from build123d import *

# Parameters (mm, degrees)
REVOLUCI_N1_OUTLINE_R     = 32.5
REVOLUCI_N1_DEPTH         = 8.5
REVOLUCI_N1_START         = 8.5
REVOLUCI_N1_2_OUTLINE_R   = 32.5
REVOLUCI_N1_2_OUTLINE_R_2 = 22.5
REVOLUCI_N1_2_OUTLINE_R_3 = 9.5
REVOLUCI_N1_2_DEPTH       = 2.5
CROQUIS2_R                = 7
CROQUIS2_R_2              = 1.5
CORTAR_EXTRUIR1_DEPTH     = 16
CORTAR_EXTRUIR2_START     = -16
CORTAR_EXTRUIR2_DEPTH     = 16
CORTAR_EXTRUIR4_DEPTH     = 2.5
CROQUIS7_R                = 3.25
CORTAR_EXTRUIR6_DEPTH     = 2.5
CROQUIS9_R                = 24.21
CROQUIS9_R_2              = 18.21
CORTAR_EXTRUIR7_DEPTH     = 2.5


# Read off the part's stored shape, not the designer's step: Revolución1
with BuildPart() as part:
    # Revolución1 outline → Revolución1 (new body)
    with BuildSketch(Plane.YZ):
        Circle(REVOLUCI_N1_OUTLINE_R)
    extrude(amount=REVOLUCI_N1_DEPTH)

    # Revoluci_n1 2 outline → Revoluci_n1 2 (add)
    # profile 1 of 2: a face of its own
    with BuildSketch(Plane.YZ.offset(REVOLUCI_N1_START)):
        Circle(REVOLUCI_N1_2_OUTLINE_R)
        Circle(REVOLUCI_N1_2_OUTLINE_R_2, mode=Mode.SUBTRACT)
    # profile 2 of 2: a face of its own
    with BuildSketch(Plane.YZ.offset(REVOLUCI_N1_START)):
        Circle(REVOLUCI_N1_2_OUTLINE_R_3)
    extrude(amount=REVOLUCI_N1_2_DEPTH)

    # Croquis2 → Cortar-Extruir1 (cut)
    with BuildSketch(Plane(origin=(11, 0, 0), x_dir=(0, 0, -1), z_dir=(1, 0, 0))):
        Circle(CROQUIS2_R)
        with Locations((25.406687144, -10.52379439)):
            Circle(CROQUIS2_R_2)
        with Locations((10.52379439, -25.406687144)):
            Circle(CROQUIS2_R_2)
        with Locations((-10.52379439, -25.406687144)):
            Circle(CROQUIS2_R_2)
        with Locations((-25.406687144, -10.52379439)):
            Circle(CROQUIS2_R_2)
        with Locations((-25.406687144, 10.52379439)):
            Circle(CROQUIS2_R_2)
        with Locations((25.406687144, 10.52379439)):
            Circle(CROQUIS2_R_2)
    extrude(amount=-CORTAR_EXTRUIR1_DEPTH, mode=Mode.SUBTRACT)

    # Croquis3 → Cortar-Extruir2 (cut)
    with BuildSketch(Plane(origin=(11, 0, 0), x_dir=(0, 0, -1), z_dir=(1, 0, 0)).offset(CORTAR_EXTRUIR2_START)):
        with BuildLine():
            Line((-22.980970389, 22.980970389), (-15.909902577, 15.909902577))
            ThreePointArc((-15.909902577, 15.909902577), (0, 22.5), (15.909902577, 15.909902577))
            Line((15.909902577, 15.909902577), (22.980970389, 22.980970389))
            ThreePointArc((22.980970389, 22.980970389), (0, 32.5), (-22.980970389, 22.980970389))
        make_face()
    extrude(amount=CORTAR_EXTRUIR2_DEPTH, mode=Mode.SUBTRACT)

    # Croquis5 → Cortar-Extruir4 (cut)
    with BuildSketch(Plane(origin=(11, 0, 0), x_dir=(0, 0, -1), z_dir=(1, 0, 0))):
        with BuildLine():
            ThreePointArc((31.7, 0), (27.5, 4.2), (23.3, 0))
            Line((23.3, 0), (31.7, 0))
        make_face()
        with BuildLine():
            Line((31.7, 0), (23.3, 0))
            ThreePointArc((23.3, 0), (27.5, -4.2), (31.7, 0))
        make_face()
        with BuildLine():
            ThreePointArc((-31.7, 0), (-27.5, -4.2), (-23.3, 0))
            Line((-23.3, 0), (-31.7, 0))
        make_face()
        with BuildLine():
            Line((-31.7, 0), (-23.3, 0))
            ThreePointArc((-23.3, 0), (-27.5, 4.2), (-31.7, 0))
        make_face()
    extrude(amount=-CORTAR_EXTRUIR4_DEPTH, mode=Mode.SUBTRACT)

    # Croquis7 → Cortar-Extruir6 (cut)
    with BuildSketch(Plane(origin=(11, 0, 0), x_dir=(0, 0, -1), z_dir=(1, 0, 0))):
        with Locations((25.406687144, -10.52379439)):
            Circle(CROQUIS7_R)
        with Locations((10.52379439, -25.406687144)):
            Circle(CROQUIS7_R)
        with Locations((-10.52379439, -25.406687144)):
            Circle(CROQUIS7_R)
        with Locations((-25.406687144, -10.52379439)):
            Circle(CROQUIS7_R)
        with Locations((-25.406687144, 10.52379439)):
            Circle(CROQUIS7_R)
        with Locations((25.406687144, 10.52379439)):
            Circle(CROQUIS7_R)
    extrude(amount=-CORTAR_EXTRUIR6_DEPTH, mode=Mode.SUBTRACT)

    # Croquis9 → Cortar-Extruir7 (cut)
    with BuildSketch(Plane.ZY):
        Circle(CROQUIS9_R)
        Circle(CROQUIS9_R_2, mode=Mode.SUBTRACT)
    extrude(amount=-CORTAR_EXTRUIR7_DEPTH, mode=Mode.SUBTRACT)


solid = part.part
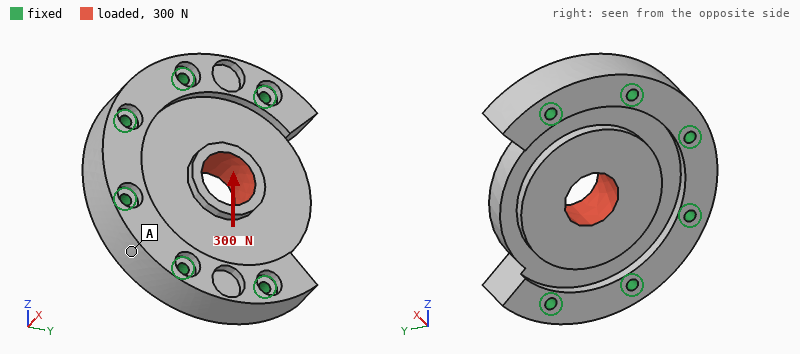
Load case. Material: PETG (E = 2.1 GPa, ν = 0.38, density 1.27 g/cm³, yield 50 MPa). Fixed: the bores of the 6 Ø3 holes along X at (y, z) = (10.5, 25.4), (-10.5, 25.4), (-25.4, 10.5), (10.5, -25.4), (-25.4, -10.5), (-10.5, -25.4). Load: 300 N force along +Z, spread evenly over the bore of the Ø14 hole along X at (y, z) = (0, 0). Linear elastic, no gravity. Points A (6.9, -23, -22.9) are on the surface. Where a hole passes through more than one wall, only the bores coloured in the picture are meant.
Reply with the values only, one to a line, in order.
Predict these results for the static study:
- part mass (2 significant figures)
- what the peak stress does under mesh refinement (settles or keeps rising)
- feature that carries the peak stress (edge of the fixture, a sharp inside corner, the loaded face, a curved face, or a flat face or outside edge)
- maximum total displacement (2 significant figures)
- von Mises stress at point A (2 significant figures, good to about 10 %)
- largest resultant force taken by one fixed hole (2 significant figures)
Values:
30 g
keeps rising
edge of the fixture
13 µm
0.21 MPa
73 N
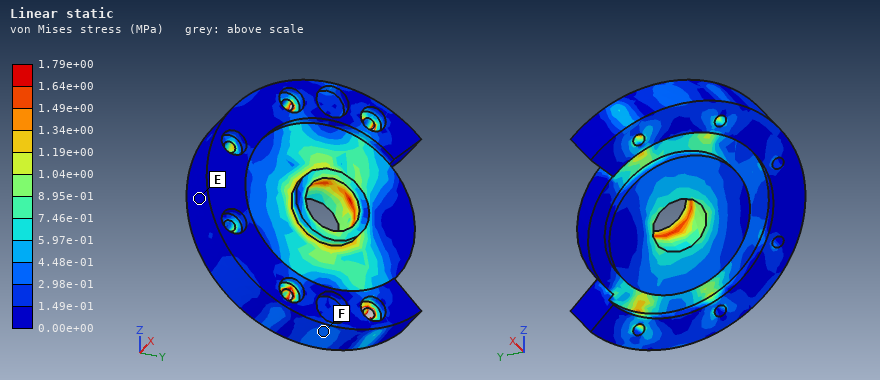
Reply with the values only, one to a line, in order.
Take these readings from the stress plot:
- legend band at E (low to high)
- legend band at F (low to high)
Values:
0.00e+00 to 1.49e-01 MPa
2.98e-01 to 4.48e-01 MPa
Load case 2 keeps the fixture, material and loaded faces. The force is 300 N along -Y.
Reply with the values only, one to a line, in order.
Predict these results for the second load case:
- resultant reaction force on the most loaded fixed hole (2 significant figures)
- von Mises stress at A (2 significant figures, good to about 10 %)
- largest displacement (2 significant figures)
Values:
77 N
0.33 MPa
22 µm
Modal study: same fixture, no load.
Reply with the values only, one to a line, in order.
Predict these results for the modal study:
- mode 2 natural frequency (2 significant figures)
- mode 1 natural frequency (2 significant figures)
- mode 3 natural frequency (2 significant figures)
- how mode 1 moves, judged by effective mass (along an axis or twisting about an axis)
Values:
5700 Hz
3100 Hz
7200 Hz
along X
